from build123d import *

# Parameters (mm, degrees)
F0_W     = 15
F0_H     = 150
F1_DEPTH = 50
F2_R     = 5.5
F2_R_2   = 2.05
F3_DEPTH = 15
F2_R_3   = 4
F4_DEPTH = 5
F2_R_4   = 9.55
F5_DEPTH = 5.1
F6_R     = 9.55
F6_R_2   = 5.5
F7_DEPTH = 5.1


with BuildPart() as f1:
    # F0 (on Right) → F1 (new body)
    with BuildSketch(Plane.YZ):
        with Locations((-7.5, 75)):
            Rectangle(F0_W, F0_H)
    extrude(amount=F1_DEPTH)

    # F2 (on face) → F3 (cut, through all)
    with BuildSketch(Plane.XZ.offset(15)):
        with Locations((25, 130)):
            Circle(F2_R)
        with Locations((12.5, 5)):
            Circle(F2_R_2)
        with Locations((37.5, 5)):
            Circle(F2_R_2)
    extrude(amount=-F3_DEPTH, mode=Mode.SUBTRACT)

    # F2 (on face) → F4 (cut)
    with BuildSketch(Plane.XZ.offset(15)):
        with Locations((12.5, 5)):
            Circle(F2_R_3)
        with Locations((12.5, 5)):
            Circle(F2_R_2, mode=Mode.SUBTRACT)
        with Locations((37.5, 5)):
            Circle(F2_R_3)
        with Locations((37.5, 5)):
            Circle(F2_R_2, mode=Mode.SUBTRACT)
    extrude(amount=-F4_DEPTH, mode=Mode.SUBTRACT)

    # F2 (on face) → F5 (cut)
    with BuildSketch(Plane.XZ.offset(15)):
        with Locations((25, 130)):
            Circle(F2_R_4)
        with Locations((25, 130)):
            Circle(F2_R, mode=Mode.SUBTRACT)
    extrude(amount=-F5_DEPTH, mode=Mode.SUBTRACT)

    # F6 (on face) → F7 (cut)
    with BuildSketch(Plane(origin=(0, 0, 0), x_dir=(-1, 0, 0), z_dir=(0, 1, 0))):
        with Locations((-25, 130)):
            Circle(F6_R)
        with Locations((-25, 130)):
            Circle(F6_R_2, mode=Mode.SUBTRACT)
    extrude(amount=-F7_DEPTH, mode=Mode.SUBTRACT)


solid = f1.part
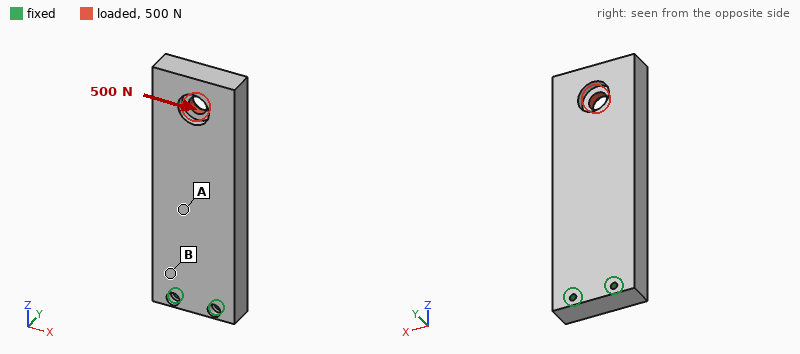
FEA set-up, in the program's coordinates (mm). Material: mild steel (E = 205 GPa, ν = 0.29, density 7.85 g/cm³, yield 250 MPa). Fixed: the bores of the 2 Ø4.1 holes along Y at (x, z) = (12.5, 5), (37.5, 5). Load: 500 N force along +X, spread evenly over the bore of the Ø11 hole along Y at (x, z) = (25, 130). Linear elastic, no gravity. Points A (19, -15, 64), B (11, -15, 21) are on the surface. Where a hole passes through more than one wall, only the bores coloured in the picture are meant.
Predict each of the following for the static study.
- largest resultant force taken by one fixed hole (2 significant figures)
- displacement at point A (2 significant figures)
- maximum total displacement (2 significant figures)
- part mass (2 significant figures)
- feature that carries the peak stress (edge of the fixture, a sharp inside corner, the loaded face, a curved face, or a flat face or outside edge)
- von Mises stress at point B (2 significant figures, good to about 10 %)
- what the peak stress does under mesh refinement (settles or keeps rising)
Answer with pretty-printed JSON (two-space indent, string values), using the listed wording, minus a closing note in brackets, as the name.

{
  "largest resultant force taken by one fixed hole": "2.3 kN",
  "displacement at point A": "6.3 µm",
  "maximum total displacement": "22 µm",
  "part mass": "850 g",
  "feature that carries the peak stress": "edge of the fixture",
  "von Mises stress at point B": "4.8 MPa",
  "what the peak stress does under mesh refinement": "keeps rising"
}
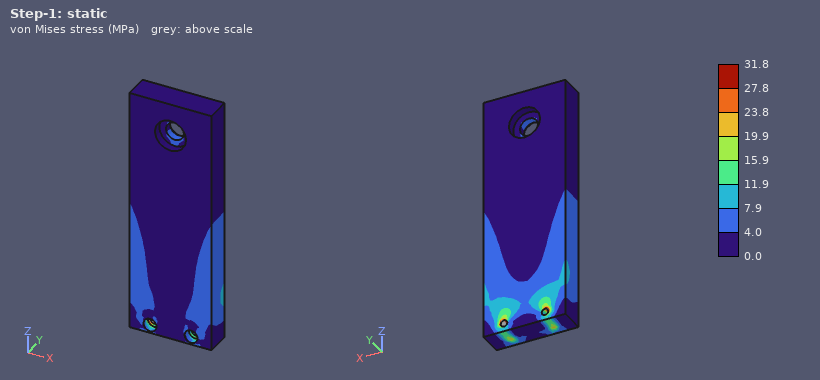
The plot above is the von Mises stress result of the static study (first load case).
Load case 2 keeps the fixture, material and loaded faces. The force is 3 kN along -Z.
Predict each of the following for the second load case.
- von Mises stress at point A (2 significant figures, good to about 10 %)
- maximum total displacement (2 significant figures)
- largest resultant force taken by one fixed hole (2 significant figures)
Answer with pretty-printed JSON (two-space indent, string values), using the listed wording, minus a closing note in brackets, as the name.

{
  "von Mises stress at point A": "4.0 MPa",
  "maximum total displacement": "9.8 µm",
  "largest resultant force taken by one fixed hole": "1.5 kN"
}
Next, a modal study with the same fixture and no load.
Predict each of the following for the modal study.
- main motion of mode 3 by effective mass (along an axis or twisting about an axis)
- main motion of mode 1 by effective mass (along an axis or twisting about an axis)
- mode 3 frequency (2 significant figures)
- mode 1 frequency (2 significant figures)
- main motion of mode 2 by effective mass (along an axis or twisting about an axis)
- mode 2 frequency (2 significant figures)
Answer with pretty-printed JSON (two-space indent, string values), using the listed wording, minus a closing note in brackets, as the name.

{
  "main motion of mode 3 by effective mass": "twisting about Z",
  "main motion of mode 1 by effective mass": "along Y",
  "mode 3 frequency": "2900 Hz",
  "mode 1 frequency": "490 Hz",
  "main motion of mode 2 by effective mass": "along X",
  "mode 2 frequency": "1500 Hz"
}
